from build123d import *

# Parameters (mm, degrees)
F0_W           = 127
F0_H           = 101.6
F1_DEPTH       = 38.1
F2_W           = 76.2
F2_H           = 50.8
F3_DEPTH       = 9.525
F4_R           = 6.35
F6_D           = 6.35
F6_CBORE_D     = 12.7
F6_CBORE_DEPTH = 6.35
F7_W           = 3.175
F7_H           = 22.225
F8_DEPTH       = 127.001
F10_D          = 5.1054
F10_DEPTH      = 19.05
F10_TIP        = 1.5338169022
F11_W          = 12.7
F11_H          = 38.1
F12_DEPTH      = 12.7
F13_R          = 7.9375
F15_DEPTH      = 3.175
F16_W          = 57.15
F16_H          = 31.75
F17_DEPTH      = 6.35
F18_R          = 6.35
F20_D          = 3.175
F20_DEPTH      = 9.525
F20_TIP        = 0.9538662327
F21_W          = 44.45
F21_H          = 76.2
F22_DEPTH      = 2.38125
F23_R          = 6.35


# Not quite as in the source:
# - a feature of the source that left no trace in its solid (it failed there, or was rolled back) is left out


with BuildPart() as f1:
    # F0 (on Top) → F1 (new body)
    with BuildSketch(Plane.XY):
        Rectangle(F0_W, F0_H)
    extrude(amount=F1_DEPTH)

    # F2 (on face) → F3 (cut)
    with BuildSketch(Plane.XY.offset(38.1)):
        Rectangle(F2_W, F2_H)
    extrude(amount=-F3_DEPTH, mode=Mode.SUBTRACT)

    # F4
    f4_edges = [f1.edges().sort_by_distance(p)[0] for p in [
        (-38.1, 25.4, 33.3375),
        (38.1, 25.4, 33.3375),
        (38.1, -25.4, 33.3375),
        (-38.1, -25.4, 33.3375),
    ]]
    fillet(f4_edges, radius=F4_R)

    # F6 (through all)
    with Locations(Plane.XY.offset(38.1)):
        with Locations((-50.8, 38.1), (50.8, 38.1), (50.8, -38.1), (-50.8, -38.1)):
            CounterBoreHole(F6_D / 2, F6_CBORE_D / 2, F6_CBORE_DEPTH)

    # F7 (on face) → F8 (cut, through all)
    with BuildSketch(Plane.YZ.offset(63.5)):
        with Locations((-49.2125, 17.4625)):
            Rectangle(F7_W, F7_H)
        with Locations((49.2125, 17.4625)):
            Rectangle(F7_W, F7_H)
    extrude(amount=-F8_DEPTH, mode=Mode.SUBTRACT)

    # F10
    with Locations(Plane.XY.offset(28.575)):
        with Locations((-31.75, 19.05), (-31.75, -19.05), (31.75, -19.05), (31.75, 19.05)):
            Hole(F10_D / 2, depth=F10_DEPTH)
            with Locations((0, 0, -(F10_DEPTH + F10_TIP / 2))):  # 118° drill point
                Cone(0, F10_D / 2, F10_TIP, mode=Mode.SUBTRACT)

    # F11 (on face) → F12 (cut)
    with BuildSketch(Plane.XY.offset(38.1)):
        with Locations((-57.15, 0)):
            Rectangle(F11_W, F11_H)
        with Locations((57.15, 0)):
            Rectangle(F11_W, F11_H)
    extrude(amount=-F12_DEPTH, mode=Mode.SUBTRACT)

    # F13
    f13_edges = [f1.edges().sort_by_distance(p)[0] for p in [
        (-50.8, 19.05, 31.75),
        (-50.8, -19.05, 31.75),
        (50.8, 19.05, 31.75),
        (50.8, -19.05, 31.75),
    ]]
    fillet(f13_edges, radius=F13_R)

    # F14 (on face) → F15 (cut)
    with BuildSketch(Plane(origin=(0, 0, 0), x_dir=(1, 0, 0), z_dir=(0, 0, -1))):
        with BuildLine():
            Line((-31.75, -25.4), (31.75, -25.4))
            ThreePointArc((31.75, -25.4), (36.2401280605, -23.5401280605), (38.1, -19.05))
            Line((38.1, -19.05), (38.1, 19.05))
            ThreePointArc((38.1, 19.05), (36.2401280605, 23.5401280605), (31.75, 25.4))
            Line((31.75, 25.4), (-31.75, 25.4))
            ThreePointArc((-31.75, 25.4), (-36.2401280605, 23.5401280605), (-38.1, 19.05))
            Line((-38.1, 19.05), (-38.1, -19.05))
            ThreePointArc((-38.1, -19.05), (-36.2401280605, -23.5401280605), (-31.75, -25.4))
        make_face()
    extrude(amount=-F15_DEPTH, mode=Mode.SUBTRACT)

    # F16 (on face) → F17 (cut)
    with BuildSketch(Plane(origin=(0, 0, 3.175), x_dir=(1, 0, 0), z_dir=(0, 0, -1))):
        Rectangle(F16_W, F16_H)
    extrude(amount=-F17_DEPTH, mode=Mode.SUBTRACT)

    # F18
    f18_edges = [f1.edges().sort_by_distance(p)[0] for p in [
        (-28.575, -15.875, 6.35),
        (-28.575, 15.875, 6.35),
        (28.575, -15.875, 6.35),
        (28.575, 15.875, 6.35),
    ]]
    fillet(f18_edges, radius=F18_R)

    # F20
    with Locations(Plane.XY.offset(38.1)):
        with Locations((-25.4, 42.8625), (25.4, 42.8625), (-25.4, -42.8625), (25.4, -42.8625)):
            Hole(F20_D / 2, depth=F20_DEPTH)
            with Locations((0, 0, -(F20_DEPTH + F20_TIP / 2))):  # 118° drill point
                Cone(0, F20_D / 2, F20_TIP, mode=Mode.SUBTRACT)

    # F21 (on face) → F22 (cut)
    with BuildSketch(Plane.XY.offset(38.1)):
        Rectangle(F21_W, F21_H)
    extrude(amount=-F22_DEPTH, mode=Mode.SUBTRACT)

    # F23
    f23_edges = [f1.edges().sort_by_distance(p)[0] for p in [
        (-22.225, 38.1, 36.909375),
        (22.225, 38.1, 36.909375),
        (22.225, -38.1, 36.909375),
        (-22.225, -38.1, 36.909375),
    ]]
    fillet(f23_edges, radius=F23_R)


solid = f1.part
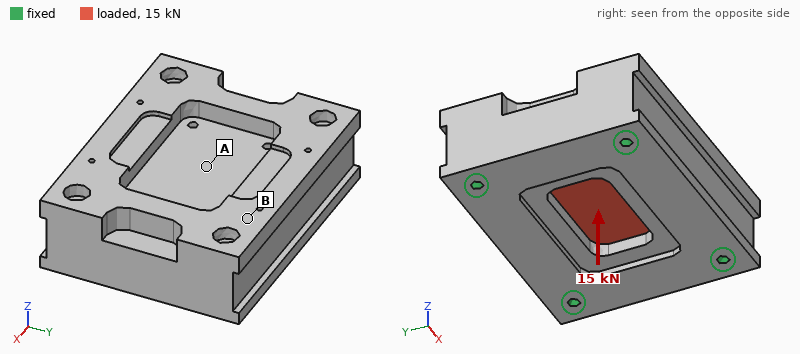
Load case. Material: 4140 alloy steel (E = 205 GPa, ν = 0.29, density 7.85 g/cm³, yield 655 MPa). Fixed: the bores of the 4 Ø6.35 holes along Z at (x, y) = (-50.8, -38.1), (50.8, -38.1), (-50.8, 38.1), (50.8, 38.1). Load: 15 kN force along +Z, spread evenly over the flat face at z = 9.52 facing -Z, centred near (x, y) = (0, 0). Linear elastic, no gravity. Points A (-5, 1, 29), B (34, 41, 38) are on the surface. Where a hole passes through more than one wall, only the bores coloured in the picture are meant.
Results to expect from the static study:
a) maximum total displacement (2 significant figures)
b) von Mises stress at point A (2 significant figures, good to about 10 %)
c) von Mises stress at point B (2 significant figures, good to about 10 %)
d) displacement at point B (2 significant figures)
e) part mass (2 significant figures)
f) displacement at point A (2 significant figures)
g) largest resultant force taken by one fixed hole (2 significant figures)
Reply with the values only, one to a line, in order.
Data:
7.2 µm
18 MPa
5.1 MPa
1.9 µm
3.1 kg
6.7 µm
3.8 kN
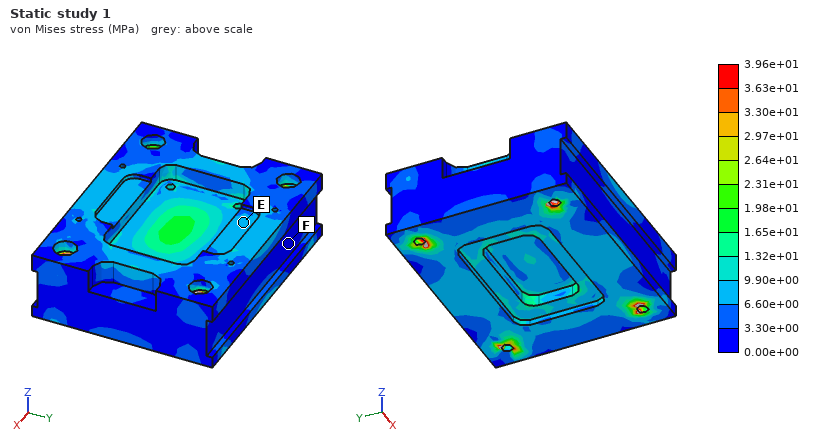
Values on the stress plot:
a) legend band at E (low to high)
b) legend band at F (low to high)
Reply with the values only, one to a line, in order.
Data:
6.60e+00 to 9.90e+00 MPa
0.00e+00 to 3.30e+00 MPa
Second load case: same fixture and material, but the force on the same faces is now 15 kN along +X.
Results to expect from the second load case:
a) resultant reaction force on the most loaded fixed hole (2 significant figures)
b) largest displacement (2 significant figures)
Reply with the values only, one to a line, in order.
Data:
4.1 kN
2.5 µm
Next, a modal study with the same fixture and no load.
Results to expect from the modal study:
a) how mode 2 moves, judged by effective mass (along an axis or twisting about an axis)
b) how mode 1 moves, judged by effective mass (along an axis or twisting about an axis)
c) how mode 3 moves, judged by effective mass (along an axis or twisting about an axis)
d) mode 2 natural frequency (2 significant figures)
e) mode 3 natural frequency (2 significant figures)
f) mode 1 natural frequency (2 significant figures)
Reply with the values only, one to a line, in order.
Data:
twisting about X
along Z
along Y
11 kHz
12 kHz
8400 Hz
